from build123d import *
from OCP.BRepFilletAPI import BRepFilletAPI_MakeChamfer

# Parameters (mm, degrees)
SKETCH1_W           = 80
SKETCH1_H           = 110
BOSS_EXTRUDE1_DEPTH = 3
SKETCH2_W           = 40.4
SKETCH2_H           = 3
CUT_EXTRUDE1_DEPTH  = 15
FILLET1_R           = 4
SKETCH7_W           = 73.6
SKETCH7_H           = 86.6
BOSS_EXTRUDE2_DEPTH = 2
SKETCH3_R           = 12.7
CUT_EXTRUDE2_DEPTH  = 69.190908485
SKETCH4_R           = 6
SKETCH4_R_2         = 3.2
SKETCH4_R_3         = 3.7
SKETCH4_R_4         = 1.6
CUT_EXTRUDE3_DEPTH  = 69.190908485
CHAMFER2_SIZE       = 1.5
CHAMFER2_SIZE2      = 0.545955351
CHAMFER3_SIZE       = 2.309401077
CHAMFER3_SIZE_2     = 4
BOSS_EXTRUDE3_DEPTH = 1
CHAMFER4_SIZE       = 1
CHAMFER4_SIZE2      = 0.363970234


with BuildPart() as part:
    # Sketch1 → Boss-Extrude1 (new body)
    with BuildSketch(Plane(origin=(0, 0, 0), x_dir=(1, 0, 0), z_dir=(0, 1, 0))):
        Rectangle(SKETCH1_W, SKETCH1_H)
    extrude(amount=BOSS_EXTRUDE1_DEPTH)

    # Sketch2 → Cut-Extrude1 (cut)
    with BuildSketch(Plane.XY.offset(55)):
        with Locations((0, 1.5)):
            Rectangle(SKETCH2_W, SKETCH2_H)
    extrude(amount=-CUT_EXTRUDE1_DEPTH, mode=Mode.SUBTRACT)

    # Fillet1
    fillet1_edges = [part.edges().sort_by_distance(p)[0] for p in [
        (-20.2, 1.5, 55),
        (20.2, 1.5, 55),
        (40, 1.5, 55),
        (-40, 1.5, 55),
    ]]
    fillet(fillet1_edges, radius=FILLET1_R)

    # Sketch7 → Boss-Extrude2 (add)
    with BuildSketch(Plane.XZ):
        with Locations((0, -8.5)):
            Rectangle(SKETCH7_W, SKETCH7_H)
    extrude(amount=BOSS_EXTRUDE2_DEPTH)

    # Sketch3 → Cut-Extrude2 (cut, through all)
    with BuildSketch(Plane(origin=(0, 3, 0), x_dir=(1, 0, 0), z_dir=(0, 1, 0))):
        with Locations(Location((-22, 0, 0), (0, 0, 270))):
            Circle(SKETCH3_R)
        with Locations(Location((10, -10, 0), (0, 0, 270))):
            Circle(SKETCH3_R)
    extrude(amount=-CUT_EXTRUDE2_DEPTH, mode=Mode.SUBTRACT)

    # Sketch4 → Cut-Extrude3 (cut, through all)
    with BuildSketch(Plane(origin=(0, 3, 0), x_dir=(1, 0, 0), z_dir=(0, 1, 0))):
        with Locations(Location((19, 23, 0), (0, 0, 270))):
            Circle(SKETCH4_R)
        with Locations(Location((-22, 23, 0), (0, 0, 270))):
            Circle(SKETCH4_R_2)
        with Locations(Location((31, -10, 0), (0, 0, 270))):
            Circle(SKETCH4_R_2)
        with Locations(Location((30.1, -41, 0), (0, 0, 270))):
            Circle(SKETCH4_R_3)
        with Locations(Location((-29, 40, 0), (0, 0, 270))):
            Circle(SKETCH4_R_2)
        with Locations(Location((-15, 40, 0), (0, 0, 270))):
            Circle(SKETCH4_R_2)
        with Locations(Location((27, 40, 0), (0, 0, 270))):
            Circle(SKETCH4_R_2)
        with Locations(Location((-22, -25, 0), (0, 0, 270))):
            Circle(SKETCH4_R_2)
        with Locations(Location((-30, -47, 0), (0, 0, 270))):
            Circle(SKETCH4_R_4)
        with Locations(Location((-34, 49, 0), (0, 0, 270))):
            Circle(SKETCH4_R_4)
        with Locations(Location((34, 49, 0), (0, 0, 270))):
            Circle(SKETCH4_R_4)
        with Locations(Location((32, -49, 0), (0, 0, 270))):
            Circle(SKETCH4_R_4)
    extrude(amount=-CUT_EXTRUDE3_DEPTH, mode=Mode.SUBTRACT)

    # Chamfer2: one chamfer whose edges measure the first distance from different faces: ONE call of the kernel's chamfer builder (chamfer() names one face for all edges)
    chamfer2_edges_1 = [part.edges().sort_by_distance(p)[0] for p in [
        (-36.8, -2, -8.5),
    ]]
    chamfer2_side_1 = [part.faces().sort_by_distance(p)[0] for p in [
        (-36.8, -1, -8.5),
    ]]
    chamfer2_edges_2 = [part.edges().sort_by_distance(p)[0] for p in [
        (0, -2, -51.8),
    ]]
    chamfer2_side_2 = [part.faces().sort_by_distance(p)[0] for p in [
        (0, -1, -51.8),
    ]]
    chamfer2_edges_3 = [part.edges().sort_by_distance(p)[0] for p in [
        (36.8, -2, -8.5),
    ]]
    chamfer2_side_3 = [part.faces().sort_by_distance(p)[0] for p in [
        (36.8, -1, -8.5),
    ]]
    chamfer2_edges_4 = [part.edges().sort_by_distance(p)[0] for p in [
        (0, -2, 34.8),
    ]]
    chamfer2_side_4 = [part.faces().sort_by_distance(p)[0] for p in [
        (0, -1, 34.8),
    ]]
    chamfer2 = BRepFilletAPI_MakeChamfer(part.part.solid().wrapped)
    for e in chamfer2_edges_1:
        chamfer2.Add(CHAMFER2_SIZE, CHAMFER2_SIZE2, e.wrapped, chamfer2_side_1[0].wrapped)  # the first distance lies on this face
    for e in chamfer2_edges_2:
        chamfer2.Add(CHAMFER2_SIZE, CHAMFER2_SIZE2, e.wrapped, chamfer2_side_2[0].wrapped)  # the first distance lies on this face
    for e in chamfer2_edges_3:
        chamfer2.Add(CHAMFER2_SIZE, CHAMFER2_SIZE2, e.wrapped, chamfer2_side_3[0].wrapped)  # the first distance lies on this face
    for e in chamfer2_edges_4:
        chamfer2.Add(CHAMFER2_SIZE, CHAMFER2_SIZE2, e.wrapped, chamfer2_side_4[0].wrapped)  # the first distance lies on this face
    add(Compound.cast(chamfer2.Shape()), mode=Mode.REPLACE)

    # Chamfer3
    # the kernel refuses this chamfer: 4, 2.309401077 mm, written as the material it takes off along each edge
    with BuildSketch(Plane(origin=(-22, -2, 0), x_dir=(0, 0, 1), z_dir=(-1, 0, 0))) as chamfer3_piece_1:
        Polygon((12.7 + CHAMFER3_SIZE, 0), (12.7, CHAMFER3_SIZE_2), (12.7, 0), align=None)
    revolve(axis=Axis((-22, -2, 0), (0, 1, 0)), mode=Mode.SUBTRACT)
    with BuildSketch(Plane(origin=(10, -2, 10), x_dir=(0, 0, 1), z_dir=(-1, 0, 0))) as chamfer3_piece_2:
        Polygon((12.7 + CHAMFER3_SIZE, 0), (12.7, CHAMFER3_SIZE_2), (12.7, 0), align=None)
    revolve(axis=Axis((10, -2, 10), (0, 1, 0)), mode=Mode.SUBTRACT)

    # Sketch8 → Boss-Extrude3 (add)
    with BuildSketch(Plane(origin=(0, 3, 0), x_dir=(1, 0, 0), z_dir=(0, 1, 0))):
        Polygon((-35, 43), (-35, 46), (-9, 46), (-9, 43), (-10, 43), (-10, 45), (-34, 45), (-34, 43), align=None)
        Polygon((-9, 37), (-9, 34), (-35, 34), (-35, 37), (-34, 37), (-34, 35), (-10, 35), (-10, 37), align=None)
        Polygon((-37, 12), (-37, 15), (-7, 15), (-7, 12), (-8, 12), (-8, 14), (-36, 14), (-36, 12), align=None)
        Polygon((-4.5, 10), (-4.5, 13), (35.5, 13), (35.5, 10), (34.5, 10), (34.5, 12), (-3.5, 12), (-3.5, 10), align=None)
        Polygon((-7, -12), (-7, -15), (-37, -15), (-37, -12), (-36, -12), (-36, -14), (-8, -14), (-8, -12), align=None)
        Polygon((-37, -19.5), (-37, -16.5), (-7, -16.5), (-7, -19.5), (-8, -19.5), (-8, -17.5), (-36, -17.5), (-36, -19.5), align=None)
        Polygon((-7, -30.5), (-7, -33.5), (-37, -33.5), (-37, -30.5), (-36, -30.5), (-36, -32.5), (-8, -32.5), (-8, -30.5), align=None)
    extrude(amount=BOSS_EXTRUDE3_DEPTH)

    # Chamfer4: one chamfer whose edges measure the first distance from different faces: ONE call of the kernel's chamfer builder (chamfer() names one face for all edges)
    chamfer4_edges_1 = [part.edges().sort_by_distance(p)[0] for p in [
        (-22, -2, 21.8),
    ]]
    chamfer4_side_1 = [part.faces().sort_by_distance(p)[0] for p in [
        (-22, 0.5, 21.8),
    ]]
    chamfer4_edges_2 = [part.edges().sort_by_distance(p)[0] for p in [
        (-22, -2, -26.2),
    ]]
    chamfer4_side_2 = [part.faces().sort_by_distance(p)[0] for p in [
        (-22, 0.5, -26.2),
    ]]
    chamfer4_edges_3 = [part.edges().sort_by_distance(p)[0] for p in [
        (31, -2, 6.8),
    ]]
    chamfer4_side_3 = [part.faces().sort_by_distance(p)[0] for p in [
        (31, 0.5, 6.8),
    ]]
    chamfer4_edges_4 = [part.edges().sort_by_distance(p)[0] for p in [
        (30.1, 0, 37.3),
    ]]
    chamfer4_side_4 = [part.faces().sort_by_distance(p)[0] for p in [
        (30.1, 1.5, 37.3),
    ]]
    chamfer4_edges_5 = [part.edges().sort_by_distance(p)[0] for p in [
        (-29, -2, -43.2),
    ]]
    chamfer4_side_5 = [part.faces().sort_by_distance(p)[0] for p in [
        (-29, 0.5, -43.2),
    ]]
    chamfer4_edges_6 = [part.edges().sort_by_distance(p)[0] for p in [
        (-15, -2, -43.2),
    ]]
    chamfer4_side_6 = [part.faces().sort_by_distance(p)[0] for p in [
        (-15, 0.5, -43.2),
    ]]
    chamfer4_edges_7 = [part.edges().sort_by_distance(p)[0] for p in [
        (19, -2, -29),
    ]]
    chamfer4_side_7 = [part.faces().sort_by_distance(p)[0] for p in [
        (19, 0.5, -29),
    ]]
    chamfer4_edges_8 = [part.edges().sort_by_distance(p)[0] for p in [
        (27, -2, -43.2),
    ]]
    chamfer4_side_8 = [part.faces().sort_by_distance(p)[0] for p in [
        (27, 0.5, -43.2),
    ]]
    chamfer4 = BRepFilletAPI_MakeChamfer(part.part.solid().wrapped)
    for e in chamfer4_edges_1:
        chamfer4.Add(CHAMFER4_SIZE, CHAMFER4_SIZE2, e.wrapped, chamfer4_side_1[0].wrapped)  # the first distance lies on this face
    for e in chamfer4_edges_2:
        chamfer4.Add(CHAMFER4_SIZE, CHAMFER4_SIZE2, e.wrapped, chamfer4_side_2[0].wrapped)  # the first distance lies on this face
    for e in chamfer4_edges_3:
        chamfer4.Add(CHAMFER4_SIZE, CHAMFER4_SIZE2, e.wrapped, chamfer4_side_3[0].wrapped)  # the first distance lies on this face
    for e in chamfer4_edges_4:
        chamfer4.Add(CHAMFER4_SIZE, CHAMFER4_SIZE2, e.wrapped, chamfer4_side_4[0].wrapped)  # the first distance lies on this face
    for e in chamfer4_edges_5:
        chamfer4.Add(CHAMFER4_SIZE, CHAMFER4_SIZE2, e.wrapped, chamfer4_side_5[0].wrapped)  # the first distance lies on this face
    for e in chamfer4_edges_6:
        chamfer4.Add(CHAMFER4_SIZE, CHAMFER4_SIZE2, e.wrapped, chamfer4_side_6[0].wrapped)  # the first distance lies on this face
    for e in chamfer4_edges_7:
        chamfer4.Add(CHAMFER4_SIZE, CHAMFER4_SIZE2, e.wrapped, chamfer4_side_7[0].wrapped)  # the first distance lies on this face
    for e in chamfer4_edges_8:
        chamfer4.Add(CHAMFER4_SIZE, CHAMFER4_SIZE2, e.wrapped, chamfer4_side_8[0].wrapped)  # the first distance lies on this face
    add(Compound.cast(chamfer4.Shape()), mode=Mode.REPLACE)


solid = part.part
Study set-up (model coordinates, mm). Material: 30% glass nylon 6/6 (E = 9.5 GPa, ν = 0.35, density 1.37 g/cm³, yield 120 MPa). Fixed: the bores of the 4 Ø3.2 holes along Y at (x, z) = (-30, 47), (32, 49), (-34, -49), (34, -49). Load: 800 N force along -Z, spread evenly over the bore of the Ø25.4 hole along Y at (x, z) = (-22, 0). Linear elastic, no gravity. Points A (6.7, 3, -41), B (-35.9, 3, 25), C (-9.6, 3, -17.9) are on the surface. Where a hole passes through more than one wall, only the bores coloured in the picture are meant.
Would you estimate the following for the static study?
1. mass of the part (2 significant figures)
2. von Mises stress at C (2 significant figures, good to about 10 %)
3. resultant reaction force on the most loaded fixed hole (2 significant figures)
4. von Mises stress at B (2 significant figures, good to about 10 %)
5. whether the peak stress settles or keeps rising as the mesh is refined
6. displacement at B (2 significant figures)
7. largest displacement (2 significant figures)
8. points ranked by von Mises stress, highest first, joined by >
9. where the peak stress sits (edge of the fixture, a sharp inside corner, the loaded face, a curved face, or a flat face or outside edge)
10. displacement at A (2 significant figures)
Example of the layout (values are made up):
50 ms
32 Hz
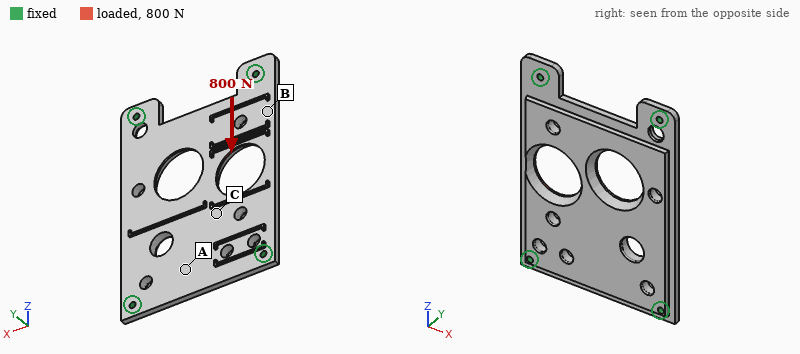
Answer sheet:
41 g
3.6 MPa
320 N
6.6 MPa
keeps rising
48 µm
64 µm
B > C > A
edge of the fixture
13 µm
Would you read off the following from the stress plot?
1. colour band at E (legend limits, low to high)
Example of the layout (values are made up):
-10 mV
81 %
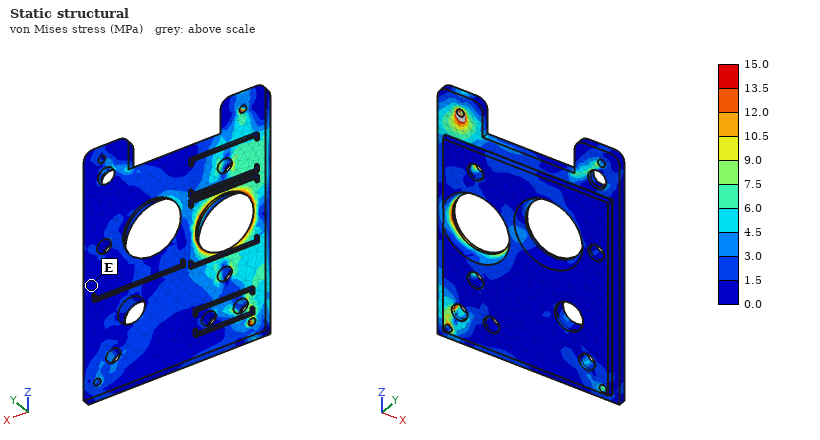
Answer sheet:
0.0 to 1.5 MPa
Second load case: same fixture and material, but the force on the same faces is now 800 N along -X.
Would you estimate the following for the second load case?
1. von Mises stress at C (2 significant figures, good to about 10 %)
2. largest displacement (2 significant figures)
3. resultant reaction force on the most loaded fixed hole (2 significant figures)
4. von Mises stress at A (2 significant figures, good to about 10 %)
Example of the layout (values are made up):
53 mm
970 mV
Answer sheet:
7.4 MPa
0.20 mm
310 N
3.2 MPa
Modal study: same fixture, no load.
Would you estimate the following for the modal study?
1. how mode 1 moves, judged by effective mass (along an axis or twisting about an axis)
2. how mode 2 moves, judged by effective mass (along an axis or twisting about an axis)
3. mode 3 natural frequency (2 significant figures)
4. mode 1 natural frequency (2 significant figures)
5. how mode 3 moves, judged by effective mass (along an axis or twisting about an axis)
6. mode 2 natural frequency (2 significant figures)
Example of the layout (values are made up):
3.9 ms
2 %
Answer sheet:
along Y
twisting about Z
2100 Hz
860 Hz
twisting about X
1500 Hz
